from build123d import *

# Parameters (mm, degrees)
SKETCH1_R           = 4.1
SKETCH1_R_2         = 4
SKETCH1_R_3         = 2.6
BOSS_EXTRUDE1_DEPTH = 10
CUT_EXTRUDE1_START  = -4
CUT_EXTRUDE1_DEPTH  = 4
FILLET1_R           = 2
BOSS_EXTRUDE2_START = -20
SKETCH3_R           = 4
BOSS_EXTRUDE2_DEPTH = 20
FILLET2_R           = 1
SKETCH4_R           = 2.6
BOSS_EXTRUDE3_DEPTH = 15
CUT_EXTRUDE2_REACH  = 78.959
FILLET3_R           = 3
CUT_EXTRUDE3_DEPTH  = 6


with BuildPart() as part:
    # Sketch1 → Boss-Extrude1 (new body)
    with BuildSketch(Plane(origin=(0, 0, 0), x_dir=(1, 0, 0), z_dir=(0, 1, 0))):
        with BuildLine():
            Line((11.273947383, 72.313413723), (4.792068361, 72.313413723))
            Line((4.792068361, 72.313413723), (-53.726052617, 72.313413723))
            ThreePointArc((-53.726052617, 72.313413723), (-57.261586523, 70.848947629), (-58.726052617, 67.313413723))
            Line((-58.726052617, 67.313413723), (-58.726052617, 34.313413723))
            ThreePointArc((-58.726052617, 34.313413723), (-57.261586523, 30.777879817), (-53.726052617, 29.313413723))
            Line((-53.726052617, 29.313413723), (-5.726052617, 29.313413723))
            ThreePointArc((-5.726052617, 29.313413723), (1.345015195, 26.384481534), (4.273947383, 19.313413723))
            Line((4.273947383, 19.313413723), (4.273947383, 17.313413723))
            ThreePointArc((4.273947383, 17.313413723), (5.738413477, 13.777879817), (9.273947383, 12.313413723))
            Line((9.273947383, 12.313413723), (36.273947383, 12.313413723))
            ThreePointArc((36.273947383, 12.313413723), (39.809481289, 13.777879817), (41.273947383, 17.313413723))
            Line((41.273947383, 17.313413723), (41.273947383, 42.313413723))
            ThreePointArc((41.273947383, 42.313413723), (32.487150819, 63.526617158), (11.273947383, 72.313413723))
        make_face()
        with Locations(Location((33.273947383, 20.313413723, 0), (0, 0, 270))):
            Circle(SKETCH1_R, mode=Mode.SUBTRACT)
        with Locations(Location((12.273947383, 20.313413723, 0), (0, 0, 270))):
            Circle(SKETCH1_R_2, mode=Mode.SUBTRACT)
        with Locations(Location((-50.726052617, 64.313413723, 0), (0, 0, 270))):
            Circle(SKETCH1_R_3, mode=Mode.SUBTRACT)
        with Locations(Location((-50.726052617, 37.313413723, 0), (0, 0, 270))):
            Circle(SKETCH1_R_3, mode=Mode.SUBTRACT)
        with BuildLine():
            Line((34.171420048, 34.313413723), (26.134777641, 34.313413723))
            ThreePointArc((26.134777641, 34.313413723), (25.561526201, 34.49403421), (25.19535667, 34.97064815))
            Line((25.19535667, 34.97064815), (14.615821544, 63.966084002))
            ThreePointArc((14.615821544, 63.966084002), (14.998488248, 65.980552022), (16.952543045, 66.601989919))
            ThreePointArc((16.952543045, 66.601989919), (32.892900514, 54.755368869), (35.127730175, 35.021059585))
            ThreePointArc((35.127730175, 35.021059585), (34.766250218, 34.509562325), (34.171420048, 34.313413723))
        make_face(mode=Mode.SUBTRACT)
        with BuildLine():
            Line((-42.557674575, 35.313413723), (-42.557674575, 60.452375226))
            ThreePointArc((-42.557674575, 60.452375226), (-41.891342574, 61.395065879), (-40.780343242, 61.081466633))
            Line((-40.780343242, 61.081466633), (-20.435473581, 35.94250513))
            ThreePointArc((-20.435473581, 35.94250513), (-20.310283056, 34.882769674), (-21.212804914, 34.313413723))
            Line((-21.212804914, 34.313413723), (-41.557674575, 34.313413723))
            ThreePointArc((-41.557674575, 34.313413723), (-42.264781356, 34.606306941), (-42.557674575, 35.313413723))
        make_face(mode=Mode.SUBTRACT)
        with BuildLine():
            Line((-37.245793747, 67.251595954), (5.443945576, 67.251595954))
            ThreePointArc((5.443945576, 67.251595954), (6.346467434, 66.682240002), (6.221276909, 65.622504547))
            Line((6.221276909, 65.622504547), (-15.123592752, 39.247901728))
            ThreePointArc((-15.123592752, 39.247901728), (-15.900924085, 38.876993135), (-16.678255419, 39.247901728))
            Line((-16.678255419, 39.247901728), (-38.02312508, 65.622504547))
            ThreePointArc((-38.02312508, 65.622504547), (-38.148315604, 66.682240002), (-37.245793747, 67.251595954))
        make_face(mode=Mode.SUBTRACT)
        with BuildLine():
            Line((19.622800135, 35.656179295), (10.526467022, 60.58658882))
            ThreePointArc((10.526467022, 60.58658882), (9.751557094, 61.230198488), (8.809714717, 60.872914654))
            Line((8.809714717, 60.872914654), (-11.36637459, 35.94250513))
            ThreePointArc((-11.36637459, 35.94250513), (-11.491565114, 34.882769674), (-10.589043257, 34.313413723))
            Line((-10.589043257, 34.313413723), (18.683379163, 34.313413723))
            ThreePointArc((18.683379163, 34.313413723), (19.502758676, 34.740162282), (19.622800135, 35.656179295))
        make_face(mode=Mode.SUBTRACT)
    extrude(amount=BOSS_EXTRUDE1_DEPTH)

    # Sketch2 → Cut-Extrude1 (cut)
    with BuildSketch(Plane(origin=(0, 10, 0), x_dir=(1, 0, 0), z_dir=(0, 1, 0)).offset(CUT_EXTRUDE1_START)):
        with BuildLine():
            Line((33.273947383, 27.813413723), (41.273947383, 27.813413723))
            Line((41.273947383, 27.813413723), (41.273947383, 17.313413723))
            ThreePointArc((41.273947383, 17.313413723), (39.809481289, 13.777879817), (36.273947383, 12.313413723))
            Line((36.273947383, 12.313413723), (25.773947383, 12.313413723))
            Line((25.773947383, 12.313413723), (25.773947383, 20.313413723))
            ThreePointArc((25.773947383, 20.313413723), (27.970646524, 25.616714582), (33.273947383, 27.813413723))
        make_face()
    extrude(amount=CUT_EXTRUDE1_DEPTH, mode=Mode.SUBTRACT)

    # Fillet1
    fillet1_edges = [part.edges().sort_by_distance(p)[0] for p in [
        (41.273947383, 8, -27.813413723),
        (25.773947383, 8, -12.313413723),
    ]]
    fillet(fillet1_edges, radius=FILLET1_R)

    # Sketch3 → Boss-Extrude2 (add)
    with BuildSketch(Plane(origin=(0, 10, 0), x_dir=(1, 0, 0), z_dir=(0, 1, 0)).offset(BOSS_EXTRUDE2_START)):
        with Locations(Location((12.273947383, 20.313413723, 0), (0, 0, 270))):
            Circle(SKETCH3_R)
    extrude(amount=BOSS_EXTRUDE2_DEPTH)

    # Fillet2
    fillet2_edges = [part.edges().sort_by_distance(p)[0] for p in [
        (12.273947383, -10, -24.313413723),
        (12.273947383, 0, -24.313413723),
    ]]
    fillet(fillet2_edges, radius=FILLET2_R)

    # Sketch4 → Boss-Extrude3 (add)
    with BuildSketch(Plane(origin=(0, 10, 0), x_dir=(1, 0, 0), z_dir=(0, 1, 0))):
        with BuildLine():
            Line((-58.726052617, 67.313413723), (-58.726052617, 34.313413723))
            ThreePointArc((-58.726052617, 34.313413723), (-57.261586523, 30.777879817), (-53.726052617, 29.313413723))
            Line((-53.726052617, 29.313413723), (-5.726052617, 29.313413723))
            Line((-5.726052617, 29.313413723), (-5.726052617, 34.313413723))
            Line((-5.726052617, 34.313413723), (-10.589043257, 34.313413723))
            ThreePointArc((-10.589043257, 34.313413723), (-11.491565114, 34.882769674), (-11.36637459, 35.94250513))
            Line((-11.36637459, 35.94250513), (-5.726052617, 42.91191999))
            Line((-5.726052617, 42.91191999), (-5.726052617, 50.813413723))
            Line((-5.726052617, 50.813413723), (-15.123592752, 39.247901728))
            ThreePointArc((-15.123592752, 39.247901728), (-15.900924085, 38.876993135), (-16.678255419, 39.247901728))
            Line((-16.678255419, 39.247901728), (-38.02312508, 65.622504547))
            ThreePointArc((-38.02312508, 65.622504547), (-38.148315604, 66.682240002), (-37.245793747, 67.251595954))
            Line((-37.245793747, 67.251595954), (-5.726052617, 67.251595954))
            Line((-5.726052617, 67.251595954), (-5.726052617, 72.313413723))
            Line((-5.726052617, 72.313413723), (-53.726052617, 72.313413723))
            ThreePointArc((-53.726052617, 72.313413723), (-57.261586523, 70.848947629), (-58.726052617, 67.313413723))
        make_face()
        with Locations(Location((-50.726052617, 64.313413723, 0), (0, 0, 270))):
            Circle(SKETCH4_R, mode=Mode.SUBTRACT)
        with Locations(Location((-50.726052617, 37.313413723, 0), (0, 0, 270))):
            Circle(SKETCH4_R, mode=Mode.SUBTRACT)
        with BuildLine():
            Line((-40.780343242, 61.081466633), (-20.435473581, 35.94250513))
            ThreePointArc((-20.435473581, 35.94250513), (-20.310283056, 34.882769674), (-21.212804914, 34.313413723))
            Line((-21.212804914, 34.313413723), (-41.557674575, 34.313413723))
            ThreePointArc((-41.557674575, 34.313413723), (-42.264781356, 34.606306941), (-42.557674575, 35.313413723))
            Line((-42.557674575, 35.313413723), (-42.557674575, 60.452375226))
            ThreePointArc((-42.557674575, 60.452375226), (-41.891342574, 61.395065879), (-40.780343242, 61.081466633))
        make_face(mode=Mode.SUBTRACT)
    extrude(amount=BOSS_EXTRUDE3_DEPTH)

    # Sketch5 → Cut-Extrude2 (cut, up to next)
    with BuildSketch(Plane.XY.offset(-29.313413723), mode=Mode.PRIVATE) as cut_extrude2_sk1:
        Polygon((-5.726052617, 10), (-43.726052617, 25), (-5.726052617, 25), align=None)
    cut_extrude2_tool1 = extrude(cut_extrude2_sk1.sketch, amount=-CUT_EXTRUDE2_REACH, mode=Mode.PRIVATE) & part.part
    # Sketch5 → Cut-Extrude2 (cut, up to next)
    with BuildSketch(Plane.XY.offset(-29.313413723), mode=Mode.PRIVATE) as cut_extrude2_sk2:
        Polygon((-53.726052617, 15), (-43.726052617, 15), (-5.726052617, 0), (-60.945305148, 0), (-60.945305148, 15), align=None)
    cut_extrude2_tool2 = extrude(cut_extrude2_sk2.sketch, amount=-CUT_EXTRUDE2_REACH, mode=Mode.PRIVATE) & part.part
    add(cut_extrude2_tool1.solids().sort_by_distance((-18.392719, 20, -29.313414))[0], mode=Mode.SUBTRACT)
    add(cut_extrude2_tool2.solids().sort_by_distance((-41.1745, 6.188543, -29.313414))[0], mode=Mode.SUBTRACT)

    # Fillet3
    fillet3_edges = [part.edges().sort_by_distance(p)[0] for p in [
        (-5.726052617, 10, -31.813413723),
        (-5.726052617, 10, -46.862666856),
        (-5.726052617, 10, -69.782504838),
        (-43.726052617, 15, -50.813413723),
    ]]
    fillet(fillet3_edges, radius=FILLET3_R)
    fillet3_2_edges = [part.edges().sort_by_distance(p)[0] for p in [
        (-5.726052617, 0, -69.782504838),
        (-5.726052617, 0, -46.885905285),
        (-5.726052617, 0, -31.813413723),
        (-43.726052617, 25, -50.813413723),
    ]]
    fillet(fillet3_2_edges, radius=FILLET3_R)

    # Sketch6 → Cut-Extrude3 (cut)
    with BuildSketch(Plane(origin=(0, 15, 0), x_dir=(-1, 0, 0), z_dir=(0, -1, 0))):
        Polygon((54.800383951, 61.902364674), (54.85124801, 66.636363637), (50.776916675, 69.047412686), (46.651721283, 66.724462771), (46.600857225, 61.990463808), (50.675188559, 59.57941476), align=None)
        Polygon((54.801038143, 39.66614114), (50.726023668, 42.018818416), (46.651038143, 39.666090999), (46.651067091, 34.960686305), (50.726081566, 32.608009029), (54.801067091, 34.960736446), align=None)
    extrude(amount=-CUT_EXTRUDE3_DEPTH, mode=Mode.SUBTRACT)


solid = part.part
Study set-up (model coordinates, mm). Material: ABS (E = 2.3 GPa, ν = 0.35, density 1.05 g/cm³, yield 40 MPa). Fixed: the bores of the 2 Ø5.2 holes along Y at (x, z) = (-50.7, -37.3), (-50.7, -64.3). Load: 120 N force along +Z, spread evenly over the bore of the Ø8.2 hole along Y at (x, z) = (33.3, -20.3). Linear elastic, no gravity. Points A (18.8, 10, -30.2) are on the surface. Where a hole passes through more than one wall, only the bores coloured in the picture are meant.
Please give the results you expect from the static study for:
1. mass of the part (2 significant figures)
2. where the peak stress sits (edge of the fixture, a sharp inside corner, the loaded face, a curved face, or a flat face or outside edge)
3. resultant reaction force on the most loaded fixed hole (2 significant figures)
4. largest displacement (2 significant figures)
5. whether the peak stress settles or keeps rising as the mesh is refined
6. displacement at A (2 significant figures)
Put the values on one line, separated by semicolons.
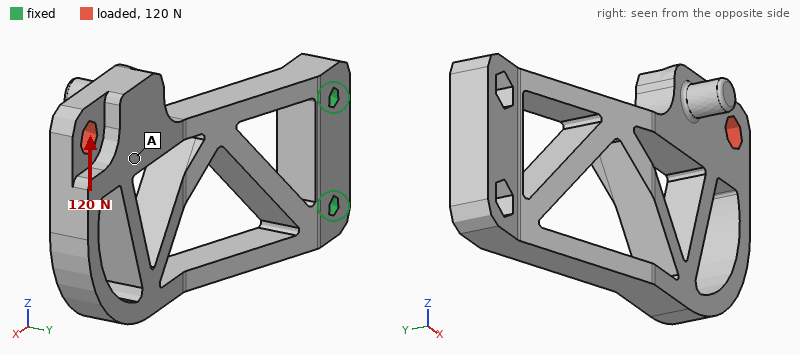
28 g; edge of the fixture; 330 N; 1.4 mm; keeps rising; 0.88 mm
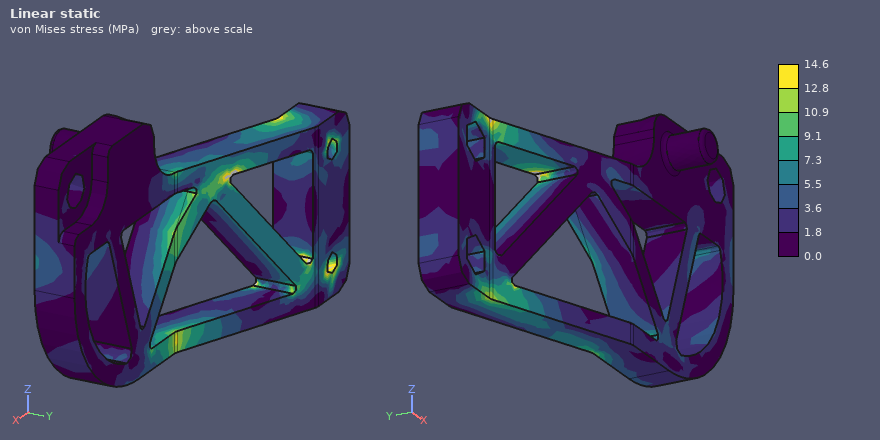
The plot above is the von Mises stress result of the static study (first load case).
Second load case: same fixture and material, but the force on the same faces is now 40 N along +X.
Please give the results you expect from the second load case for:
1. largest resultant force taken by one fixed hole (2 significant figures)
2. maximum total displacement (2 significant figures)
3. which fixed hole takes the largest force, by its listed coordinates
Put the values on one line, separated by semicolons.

57 N; 1.2 mm; (-50.7, -37.3)
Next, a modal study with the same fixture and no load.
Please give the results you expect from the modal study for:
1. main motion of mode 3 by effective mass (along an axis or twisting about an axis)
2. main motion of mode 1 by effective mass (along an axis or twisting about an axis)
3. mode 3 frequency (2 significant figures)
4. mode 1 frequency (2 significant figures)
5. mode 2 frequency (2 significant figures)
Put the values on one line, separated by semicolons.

along Z; along Y; 660 Hz; 150 Hz; 430 Hz
